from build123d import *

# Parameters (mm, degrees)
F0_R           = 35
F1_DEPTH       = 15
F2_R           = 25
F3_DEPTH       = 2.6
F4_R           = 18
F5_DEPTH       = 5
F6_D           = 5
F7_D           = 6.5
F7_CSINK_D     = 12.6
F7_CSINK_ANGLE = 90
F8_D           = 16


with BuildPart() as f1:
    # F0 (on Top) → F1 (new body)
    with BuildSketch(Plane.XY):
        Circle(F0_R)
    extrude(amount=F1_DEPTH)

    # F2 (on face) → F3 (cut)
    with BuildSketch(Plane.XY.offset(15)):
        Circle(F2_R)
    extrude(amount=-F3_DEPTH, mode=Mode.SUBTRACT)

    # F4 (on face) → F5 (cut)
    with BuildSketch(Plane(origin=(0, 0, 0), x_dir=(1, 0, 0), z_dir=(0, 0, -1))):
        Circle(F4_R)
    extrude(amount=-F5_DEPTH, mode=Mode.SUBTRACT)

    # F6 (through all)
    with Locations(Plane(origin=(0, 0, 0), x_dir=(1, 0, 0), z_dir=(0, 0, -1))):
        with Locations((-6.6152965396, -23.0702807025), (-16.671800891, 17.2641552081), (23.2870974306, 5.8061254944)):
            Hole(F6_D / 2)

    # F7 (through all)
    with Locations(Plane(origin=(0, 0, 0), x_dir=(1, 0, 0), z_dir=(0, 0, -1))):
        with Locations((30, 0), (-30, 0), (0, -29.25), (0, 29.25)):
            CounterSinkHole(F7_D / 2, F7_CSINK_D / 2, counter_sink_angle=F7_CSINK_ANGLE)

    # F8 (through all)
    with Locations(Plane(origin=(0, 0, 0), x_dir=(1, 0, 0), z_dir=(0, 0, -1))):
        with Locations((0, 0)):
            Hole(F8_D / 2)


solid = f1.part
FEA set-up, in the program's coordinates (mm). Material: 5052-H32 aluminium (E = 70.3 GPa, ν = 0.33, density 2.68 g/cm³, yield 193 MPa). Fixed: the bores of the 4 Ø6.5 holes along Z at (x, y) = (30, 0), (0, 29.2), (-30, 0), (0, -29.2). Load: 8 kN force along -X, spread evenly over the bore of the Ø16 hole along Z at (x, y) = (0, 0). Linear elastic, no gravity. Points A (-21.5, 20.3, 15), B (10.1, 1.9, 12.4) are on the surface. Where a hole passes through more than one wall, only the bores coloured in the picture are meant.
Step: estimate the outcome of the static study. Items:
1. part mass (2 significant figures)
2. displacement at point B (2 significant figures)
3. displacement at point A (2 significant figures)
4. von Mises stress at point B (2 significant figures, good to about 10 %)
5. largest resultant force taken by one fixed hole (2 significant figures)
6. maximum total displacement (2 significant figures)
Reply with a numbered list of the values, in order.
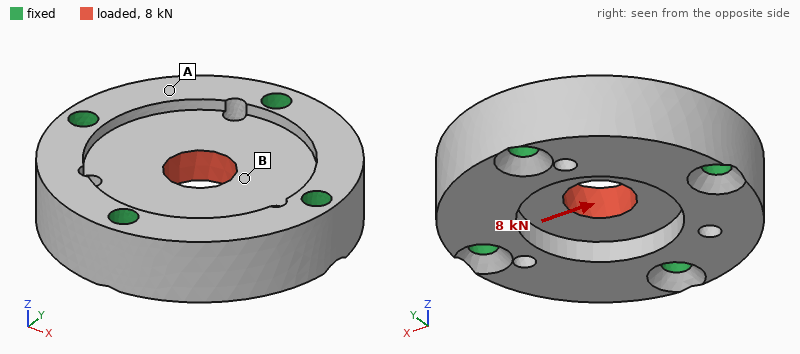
1. 110 g
2. 5.5 µm
3. 2.6 µm
4. 24 MPa
5. 2.5 kN
6. 6.7 µm
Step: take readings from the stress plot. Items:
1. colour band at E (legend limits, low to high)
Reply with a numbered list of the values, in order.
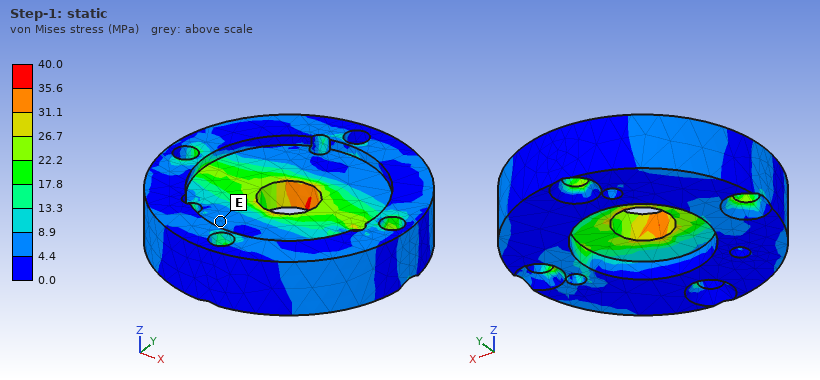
1. 4.4 to 8.9 MPa
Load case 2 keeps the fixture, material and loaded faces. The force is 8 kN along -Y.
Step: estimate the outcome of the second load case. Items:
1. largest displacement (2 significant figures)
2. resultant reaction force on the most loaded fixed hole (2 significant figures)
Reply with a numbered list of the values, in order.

1. 6.7 µm
2. 2.6 kN
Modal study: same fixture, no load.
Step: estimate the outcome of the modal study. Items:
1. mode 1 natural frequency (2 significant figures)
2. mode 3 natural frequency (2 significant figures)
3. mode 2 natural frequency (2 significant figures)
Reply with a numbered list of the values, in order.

1. 21 kHz
2. 23 kHz
3. 22 kHz
